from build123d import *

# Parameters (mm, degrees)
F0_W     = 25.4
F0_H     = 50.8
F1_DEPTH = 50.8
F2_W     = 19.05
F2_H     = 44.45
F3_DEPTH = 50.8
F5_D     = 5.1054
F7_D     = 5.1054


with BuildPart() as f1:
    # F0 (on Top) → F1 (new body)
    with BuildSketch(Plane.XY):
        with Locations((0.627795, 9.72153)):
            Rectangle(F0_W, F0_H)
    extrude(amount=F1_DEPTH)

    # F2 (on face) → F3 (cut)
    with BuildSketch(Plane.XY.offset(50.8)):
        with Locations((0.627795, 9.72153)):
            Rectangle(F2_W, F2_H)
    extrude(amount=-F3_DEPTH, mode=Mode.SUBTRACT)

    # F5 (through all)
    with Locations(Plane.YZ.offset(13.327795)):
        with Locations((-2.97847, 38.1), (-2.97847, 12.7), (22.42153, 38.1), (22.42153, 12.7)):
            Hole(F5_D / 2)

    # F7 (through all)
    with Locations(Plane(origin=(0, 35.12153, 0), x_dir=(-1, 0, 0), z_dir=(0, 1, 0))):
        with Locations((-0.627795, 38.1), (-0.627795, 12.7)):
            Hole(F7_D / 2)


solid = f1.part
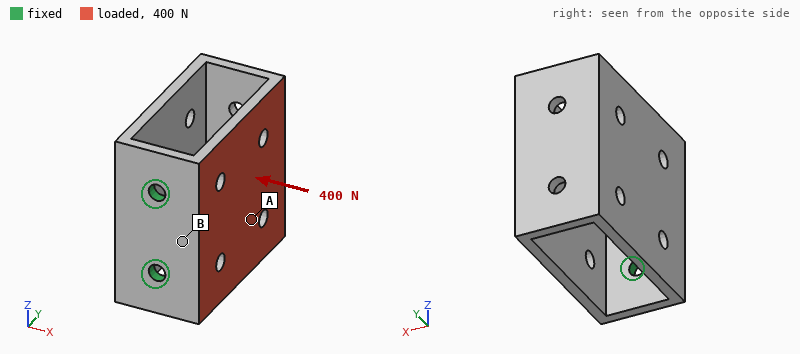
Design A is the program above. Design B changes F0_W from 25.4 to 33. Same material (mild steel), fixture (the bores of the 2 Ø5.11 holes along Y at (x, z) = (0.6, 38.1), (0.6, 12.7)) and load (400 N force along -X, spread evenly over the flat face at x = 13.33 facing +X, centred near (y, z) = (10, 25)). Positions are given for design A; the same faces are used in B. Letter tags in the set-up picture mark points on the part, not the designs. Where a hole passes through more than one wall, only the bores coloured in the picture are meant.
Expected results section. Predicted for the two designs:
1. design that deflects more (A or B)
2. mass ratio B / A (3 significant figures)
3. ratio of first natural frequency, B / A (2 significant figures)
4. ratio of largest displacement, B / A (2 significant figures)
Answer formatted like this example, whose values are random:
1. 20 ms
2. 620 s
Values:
1. A
2. 1.87
3. 0.87
4. 0.73
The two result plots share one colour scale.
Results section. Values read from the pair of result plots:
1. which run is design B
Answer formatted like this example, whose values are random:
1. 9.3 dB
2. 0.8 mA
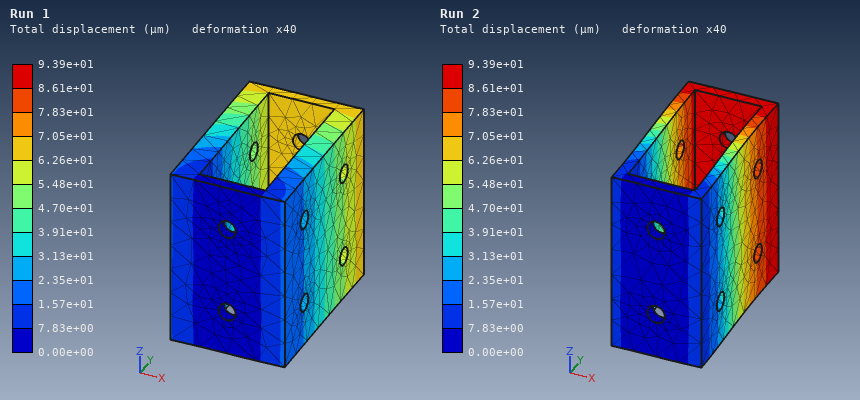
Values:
1. Run 1
